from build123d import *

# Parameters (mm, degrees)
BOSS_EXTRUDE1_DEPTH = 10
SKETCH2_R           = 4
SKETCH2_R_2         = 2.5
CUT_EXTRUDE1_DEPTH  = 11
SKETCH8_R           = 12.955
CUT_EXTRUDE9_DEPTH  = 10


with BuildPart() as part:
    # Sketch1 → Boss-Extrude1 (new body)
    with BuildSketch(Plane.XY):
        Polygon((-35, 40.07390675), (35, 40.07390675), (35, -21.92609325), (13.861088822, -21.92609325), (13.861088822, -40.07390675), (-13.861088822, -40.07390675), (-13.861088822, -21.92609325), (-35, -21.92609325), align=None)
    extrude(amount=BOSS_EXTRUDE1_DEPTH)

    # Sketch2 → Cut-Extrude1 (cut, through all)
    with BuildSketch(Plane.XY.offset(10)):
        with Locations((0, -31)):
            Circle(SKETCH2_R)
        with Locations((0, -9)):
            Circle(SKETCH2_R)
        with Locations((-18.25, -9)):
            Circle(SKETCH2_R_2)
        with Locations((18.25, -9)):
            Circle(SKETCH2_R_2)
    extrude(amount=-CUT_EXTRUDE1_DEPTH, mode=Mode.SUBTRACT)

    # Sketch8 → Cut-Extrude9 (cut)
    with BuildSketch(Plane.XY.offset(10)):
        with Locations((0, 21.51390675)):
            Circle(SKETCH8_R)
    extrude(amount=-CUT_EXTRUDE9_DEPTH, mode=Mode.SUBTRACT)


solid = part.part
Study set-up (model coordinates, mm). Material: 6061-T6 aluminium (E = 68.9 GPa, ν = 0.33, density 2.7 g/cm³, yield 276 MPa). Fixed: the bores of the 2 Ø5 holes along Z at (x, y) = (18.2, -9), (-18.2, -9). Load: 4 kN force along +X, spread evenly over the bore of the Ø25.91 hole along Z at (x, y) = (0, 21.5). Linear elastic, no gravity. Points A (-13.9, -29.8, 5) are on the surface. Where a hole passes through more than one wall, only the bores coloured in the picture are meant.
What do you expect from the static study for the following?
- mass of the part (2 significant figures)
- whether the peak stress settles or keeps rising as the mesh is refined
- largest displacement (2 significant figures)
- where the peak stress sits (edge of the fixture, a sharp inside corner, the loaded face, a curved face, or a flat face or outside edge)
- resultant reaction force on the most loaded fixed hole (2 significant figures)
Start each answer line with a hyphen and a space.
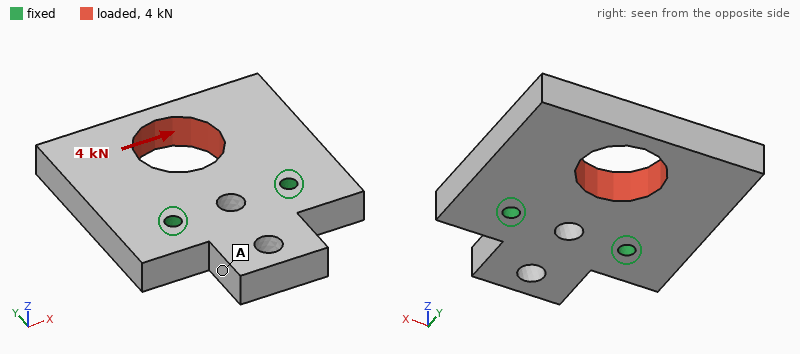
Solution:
- 110 g
- keeps rising
- 39 µm
- edge of the fixture
- 3.5 kN
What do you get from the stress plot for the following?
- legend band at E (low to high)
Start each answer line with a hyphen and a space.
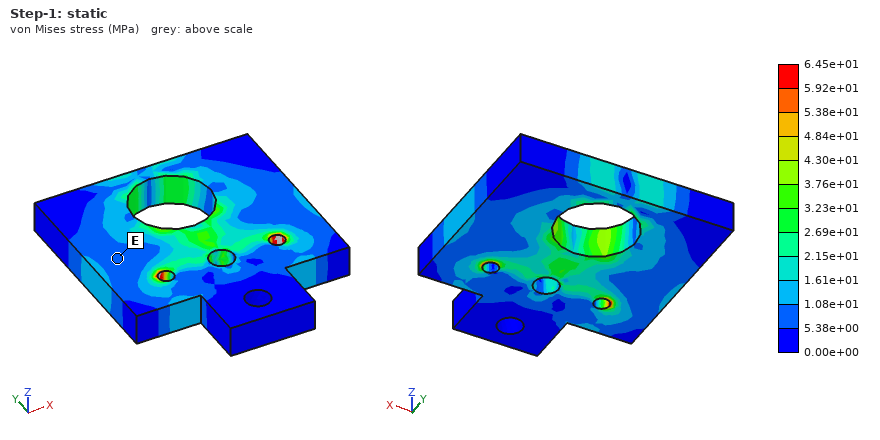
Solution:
- 5.38e+00 to 1.08e+01 MPa
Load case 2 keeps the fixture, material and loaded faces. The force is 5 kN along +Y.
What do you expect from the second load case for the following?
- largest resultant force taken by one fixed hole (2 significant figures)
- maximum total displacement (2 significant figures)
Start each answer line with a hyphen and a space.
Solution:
- 2.5 kN
- 16 µm
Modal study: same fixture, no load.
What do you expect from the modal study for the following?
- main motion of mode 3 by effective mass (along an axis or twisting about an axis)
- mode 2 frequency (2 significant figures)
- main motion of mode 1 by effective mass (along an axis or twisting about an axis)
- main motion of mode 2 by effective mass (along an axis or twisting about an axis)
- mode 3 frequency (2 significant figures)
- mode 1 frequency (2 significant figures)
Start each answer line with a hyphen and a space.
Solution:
- along X
- 4800 Hz
- along Z
- twisting about Y
- 7800 Hz
- 3000 Hz
